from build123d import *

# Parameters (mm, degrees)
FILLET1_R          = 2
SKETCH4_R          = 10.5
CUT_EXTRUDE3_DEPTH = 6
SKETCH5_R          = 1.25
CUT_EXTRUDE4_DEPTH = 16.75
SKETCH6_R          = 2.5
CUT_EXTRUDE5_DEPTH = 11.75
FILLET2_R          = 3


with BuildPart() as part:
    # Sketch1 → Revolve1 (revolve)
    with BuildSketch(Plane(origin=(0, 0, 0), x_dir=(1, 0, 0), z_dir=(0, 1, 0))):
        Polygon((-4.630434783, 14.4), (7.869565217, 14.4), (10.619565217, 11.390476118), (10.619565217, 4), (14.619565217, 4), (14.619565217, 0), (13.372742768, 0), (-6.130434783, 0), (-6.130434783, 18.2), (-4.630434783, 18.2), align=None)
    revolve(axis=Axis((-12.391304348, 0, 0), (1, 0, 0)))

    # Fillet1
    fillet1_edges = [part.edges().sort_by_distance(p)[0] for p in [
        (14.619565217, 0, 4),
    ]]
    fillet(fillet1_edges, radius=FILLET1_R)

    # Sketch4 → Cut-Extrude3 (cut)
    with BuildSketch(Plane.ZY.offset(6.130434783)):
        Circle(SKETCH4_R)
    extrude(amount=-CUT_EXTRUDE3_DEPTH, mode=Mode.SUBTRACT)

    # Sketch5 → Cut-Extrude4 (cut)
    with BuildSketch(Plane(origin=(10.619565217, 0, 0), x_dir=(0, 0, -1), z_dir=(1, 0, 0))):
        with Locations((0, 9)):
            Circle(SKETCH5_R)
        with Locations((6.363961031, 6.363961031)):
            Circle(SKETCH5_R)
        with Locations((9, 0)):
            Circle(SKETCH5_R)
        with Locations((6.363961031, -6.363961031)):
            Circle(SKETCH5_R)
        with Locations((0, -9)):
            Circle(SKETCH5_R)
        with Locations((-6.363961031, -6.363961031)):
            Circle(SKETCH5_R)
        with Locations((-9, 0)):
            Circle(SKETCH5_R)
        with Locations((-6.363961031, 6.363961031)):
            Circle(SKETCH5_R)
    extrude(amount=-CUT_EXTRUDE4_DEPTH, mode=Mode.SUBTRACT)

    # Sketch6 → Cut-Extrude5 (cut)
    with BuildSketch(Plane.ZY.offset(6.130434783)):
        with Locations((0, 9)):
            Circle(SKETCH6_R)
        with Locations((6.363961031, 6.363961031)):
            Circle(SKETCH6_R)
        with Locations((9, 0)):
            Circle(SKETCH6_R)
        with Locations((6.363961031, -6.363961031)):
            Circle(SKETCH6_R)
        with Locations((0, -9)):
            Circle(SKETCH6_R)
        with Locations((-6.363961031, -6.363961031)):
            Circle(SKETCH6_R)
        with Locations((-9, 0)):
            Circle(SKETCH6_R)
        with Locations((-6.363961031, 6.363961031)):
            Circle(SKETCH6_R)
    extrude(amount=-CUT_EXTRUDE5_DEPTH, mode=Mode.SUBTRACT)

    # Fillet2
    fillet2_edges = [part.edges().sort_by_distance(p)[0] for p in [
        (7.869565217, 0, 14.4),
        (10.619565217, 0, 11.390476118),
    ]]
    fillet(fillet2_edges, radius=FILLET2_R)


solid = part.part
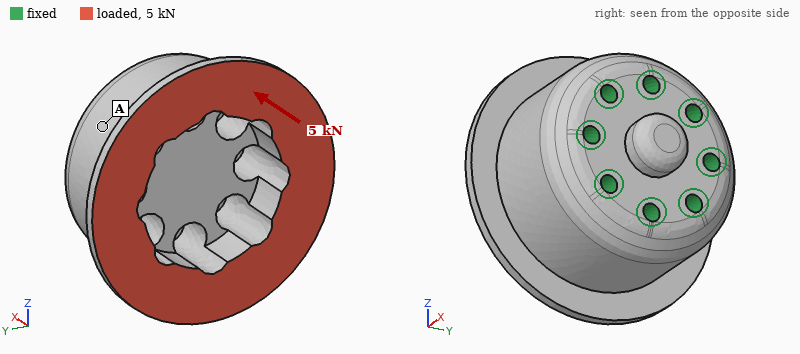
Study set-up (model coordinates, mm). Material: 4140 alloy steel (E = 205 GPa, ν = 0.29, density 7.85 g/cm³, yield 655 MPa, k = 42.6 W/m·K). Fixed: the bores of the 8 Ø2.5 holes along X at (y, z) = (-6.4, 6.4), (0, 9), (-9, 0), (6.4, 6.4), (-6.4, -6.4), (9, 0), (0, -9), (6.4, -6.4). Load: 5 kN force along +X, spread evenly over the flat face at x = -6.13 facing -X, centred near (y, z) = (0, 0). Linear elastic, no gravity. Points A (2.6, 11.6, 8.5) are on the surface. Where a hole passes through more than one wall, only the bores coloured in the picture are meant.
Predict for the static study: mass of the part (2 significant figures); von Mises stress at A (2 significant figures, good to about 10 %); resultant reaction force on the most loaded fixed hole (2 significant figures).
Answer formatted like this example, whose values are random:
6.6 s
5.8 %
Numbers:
63 g
17 MPa
630 N
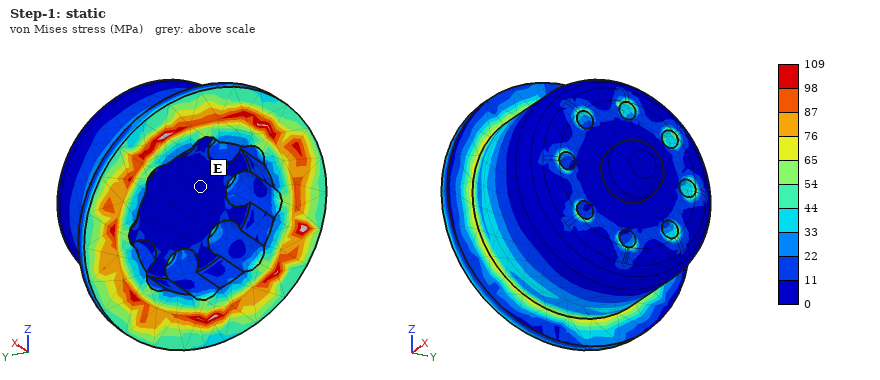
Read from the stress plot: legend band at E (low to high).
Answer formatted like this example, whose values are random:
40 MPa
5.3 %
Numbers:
0 to 11 MPa
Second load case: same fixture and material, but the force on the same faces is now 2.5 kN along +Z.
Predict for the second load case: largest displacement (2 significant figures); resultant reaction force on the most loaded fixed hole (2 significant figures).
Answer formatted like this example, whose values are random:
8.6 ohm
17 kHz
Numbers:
8.6 µm
770 N
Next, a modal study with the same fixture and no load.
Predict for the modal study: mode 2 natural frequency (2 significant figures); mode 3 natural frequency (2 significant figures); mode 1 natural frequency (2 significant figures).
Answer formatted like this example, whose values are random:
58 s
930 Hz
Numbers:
29 kHz
31 kHz
29 kHz
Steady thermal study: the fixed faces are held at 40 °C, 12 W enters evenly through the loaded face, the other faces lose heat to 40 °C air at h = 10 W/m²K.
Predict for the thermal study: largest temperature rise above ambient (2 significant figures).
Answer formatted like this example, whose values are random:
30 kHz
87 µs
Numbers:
16 K
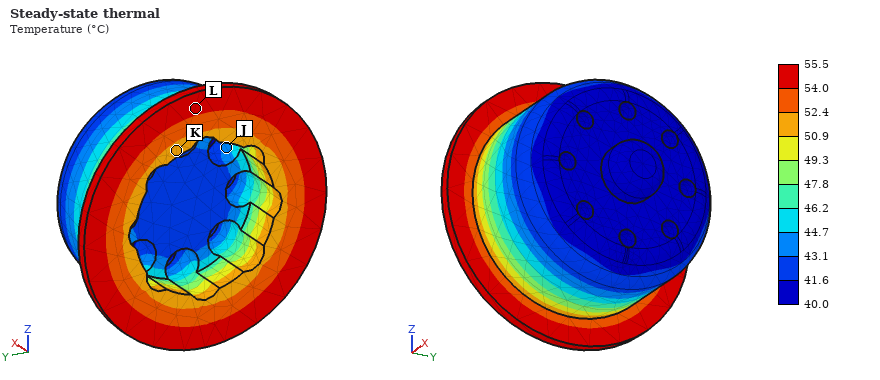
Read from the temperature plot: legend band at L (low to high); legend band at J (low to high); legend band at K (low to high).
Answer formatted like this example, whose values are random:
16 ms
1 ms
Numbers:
54.0 to 55.5 °C
43.1 to 44.7 °C
50.9 to 52.4 °C
